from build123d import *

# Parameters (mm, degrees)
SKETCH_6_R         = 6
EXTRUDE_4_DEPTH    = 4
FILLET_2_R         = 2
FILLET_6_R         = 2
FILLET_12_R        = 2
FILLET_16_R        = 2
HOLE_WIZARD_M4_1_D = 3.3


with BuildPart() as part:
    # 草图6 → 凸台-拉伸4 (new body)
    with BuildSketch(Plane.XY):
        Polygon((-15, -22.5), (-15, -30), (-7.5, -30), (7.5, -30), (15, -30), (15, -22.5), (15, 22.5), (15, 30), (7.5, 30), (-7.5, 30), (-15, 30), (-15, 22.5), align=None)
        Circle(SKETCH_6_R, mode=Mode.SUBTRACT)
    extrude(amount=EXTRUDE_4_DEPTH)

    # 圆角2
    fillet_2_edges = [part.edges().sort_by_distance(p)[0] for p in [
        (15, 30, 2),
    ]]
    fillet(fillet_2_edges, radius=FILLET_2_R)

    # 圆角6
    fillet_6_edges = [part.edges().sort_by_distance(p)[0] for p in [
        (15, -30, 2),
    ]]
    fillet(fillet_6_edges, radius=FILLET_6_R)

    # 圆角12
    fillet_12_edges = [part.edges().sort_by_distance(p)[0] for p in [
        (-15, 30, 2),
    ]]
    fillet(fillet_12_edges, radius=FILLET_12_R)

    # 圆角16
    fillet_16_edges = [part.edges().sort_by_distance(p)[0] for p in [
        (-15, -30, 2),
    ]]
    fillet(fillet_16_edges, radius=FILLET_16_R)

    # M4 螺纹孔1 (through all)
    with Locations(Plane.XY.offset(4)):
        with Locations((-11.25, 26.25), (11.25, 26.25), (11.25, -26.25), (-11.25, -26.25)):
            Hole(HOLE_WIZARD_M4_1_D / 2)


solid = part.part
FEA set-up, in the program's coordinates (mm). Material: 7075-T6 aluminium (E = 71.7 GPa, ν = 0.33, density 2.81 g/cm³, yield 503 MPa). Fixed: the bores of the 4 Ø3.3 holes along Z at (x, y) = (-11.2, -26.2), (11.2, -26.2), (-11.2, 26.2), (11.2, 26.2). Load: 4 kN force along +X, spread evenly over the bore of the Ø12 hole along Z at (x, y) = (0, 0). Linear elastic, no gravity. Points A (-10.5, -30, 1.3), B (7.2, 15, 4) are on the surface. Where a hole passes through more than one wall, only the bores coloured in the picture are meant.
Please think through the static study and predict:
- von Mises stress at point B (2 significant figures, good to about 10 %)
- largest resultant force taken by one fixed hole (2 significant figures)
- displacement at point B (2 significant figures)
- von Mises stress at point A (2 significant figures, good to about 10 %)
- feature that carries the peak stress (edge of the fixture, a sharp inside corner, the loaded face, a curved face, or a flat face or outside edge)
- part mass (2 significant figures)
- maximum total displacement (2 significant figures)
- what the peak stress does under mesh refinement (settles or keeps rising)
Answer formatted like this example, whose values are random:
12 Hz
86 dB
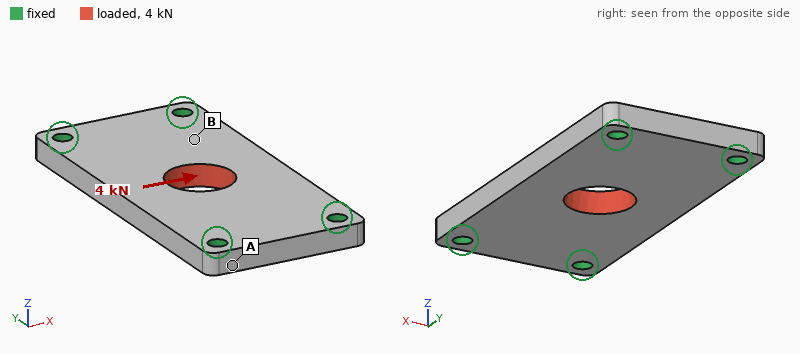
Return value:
34 MPa
1.5 kN
10 µm
18 MPa
edge of the fixture
19 g
23 µm
keeps rising
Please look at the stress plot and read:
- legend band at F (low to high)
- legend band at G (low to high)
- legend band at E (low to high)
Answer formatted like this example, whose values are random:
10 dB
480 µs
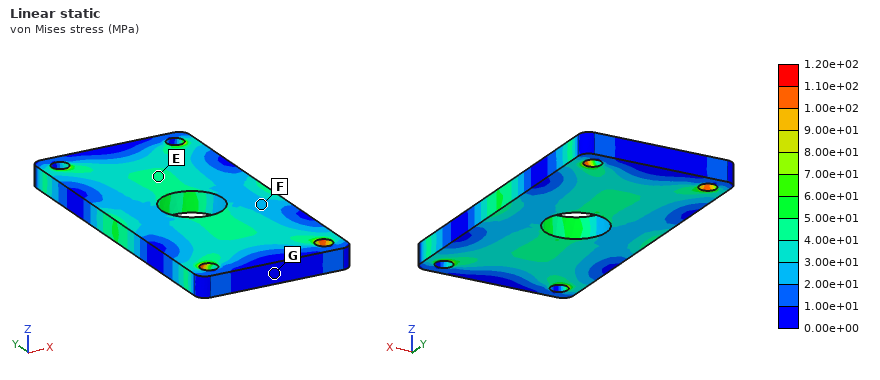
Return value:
2.00e+01 to 3.00e+01 MPa
0.00e+00 to 1.00e+01 MPa
4.00e+01 to 5.00e+01 MPa
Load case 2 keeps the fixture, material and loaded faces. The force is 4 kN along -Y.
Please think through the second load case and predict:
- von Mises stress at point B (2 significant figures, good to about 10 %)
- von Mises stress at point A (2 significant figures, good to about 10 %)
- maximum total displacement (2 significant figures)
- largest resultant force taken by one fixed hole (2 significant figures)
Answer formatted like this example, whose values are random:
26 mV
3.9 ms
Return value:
20 MPa
18 MPa
8.2 µm
1.0 kN
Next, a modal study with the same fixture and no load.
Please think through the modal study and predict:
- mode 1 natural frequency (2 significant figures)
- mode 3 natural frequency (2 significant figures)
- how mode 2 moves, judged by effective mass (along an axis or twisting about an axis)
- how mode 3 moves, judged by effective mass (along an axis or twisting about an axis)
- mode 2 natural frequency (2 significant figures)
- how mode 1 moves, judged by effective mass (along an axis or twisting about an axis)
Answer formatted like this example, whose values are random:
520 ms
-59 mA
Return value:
7100 Hz
18 kHz
twisting about Y
twisting about X
11 kHz
along Z
